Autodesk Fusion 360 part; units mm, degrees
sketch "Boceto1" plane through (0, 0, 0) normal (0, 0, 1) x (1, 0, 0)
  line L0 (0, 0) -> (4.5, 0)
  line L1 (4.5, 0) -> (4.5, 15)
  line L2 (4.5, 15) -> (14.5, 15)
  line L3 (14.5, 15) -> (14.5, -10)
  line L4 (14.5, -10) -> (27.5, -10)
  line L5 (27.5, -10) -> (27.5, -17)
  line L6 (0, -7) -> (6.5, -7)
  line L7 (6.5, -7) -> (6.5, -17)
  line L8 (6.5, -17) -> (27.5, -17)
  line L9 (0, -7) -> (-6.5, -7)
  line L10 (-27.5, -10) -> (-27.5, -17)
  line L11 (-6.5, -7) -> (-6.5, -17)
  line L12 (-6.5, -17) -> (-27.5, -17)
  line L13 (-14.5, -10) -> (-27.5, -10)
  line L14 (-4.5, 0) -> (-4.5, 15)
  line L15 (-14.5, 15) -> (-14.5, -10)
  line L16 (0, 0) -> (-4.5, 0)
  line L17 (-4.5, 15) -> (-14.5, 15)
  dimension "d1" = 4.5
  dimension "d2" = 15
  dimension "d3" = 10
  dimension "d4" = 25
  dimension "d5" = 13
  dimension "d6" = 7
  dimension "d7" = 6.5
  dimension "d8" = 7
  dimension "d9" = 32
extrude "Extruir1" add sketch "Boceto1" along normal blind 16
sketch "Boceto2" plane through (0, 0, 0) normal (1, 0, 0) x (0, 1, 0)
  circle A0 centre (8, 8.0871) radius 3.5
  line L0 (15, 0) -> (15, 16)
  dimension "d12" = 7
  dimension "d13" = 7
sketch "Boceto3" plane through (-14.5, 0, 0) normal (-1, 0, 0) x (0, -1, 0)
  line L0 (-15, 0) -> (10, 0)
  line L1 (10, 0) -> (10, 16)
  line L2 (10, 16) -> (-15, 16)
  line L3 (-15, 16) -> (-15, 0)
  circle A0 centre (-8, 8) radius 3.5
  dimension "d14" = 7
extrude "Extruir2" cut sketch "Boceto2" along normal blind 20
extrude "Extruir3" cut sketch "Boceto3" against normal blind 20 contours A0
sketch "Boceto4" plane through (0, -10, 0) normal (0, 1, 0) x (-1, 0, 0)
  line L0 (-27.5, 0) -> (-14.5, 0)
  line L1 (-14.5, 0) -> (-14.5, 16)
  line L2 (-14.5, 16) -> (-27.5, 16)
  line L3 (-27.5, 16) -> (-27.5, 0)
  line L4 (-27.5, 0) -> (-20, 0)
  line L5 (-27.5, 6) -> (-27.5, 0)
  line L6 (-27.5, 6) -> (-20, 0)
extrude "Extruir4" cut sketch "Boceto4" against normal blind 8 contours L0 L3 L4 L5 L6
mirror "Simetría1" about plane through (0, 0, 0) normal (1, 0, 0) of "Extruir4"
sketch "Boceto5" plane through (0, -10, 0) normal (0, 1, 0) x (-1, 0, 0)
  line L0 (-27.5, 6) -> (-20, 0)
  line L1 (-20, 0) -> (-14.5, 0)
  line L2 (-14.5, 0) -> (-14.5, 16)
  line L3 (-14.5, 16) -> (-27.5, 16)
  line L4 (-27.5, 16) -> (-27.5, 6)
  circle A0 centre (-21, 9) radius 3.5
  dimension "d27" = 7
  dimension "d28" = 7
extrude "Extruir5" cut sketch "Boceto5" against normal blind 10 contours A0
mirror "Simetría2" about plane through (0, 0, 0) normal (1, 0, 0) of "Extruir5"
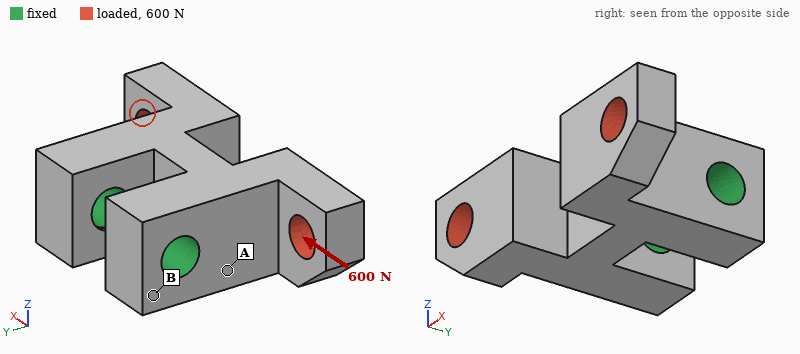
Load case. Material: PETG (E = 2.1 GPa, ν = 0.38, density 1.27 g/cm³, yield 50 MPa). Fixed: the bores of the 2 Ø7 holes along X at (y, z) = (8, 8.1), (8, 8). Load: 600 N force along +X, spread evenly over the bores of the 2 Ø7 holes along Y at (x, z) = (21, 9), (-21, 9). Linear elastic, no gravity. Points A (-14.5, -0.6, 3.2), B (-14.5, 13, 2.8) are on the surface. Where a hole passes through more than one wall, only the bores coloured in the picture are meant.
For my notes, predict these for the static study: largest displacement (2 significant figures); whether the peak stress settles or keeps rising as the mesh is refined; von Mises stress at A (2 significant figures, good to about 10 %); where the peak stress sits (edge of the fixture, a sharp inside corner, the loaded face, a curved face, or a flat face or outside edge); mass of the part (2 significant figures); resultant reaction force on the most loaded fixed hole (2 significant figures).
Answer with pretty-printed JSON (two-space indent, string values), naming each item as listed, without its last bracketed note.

{
  "largest displacement": "0.40 mm",
  "whether the peak stress settles or keeps rising as the mesh is refined": "keeps rising",
  "von Mises stress at A": "6.8 MPa",
  "where the peak stress sits": "edge of the fixture",
  "mass of the part": "15 g",
  "resultant reaction force on the most loaded fixed hole": "440 N"
}
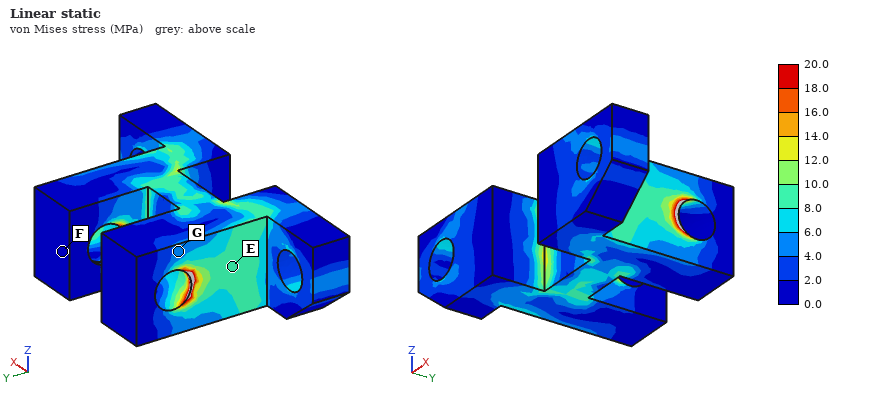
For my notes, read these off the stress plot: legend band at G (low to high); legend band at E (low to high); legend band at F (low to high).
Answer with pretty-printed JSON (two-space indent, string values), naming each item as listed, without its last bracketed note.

{
  "legend band at G": "4.0 to 6.0 MPa",
  "legend band at E": "8.0 to 10.0 MPa",
  "legend band at F": "0.0 to 2.0 MPa"
}
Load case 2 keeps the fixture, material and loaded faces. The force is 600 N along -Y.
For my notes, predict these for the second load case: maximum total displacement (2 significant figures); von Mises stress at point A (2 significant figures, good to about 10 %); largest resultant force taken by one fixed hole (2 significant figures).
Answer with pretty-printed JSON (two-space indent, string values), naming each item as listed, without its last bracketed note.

{
  "maximum total displacement": "0.72 mm",
  "von Mises stress at point A": "9.8 MPa",
  "largest resultant force taken by one fixed hole": "380 N"
}
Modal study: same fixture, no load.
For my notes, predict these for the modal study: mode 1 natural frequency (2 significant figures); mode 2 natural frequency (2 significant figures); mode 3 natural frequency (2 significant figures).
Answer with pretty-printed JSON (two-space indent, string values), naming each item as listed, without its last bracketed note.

{
  "mode 1 natural frequency": "2800 Hz",
  "mode 2 natural frequency": "2900 Hz",
  "mode 3 natural frequency": "2900 Hz"
}
